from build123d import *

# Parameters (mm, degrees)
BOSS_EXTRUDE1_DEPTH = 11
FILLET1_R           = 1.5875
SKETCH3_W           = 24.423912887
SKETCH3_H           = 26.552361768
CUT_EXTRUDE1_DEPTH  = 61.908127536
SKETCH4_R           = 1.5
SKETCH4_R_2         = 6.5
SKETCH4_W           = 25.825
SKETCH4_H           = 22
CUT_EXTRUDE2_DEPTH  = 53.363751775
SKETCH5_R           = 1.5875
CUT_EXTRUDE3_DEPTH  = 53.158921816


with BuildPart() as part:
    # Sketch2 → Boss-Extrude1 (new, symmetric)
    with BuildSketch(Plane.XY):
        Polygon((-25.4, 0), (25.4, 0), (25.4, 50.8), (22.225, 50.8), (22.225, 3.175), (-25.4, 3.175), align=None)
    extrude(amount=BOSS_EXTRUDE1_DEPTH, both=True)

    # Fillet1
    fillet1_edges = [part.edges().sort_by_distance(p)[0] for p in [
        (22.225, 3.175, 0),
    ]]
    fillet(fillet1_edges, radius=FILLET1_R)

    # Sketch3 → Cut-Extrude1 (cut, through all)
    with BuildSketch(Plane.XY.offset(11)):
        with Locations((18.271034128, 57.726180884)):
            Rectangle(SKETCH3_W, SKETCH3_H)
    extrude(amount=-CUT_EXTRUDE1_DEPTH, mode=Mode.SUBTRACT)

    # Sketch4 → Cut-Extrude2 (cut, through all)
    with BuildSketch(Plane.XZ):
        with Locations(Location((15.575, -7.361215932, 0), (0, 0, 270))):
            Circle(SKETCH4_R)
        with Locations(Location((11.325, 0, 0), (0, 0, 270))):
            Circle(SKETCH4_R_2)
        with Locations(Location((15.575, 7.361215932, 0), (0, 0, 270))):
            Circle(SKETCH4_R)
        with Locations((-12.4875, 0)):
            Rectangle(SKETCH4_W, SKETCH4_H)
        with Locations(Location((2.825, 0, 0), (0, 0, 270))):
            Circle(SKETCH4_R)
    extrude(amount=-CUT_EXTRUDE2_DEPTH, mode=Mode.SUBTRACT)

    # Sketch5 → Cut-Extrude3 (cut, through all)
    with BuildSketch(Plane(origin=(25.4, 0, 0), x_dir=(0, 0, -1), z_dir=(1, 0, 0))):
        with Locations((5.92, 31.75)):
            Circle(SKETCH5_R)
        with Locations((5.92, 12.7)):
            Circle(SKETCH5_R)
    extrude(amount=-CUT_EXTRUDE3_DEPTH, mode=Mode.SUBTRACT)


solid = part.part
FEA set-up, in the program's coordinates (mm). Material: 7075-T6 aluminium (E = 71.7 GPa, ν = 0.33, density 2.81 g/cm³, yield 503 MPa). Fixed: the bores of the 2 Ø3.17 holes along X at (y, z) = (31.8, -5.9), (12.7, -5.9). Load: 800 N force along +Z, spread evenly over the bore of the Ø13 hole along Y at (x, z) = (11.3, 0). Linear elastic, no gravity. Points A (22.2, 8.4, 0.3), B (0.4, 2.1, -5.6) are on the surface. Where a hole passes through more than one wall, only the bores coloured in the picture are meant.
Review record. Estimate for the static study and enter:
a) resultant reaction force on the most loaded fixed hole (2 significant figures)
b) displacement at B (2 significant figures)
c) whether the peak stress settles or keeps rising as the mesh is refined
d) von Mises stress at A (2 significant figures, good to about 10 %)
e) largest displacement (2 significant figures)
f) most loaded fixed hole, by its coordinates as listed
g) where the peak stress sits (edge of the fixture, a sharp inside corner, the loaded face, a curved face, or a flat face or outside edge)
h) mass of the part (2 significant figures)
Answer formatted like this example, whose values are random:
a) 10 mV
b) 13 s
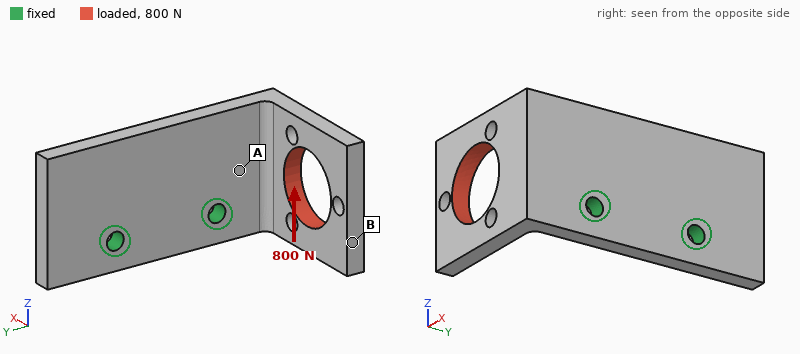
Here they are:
a) 1.2 kN
b) 0.47 mm
c) keeps rising
d) 150 MPa
e) 0.56 mm
f) (12.7, -5.9)
g) edge of the fixture
h) 12 g
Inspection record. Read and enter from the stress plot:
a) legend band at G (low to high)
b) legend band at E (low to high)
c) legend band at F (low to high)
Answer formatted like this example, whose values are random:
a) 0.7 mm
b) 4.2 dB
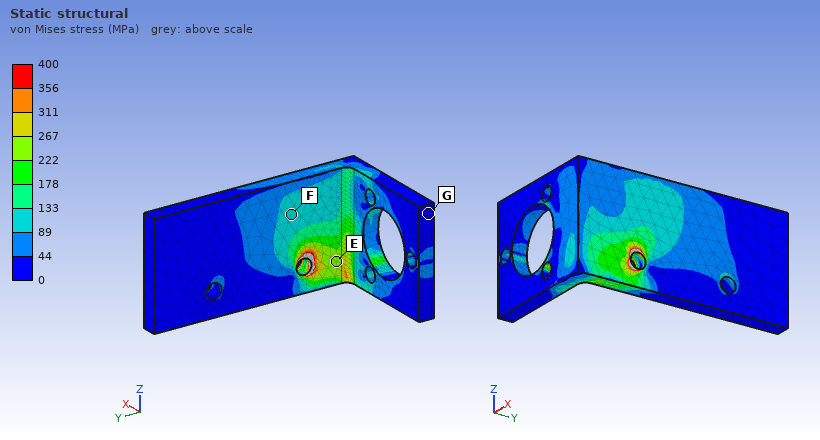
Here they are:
a) 0 to 44 MPa
b) 222 to 267 MPa
c) 89 to 133 MPa
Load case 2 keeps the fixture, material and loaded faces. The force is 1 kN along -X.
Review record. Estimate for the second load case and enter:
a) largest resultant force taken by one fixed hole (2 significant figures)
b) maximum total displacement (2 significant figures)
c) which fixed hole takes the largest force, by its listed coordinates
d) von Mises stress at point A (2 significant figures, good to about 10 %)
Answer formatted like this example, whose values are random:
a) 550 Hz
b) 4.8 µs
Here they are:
a) 1.2 kN
b) 0.56 mm
c) (12.7, -5.9)
d) 160 MPa
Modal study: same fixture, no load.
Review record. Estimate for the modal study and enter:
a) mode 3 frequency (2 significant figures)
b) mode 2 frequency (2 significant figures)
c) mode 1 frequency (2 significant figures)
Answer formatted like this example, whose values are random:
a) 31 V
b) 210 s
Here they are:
a) 7900 Hz
b) 3800 Hz
c) 2700 Hz
